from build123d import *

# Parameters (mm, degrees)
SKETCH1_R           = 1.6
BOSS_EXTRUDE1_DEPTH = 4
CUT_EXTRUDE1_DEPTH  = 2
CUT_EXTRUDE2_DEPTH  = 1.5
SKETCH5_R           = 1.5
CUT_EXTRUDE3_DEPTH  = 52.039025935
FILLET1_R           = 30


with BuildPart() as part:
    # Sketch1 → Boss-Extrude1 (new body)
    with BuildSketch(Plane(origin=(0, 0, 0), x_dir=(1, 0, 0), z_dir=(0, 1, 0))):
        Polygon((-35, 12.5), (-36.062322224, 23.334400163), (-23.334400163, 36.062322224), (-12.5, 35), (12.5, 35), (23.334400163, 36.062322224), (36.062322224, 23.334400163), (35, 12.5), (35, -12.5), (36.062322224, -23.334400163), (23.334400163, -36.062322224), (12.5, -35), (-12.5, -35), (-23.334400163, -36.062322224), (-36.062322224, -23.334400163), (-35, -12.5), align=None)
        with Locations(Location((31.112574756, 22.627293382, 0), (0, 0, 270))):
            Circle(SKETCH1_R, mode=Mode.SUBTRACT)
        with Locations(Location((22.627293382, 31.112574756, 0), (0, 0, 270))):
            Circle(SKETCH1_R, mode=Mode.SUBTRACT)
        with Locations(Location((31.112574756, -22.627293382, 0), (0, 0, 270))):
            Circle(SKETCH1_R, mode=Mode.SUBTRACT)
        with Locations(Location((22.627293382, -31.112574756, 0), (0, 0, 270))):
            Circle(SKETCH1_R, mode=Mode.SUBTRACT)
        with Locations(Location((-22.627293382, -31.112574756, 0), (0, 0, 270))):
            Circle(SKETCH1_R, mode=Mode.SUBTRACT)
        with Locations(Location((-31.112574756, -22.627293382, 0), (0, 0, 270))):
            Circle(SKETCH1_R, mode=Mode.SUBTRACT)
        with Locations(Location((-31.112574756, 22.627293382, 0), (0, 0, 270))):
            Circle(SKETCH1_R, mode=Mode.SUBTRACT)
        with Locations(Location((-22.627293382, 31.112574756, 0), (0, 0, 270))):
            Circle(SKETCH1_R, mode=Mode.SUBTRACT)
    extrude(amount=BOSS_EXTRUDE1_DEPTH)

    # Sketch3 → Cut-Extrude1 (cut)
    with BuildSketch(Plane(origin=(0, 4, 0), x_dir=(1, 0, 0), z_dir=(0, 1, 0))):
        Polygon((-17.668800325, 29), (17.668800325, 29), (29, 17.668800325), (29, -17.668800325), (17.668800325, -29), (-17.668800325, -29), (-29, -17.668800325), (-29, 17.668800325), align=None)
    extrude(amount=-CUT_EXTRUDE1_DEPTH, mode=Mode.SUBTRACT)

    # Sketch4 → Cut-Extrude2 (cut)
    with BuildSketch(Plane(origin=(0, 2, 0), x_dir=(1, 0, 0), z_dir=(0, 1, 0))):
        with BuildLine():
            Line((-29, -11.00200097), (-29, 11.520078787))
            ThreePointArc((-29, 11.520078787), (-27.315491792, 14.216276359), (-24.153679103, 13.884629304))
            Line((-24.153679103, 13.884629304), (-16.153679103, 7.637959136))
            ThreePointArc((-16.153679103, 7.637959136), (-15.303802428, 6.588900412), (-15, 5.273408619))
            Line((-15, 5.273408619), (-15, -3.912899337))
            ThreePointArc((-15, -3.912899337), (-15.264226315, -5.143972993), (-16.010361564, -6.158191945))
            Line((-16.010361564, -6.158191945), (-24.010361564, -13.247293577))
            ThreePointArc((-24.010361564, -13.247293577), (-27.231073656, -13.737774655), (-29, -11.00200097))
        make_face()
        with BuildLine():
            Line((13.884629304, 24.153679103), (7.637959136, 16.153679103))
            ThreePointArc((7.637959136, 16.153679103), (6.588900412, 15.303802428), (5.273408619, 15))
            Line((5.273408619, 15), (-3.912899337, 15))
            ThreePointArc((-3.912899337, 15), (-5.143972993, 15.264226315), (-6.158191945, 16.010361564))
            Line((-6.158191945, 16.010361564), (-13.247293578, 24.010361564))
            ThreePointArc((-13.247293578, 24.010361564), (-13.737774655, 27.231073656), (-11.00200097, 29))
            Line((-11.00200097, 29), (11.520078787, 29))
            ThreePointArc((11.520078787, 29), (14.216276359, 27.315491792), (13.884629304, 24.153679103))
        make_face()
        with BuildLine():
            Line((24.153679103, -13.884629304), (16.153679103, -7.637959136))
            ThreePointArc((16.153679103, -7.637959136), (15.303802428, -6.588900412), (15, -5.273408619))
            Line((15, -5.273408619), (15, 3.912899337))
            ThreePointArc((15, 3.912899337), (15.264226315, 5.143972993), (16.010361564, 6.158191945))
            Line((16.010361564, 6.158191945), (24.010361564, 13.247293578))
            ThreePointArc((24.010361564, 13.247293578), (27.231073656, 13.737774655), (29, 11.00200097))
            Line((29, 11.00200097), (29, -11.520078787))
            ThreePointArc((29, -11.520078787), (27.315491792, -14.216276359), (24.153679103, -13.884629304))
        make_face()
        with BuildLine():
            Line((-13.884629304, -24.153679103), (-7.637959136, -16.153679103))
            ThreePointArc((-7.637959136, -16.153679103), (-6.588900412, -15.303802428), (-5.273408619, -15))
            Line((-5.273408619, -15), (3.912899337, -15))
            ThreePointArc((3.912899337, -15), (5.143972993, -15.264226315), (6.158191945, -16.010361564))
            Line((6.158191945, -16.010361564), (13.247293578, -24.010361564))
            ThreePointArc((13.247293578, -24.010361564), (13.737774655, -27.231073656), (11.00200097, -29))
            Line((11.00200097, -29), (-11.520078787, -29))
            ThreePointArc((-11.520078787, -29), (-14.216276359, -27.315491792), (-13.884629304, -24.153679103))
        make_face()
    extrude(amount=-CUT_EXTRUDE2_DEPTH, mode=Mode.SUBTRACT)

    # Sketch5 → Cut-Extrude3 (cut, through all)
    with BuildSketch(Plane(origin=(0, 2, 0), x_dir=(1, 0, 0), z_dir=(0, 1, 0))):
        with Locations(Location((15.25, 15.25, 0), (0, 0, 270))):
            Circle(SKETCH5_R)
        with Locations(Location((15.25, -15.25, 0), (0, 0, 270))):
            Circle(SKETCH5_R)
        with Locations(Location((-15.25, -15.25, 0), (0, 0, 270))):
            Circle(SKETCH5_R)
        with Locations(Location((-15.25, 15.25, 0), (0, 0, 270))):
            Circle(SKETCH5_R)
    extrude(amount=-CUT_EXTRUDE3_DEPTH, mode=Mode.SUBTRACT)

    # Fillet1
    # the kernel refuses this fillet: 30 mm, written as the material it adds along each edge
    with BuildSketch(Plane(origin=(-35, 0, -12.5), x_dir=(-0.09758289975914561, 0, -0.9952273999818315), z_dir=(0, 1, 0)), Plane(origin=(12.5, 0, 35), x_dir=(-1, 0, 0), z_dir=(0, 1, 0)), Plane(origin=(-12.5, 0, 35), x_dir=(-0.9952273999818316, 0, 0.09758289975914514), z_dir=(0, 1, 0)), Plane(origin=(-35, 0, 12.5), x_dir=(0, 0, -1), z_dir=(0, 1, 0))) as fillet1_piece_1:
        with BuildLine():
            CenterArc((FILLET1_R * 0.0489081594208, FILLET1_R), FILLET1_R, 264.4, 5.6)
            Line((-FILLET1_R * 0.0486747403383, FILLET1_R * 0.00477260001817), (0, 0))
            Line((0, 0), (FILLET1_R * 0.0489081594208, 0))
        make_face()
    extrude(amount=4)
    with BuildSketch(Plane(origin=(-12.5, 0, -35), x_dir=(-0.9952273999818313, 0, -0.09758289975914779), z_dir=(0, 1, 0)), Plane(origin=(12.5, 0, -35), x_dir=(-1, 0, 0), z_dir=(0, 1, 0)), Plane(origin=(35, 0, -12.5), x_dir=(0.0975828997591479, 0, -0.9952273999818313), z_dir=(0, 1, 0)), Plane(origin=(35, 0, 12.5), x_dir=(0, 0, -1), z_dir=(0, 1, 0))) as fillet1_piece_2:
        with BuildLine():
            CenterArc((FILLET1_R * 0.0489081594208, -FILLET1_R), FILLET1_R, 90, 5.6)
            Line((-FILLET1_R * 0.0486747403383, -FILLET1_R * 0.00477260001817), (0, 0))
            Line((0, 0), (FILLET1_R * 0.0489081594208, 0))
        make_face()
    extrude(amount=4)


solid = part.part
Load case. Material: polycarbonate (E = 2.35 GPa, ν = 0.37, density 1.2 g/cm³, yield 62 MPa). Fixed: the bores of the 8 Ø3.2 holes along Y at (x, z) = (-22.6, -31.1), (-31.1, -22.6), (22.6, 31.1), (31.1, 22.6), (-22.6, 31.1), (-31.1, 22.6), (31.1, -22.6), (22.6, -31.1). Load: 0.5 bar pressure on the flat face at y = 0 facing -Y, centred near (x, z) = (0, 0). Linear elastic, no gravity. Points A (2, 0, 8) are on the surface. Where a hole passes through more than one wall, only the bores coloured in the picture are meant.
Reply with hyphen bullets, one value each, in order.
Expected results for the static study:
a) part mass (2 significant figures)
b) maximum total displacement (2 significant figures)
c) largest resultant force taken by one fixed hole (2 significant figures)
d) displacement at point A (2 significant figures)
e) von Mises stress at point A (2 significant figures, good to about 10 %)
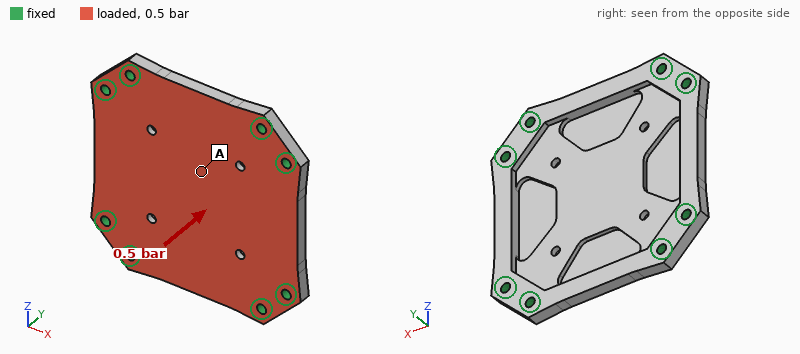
- 13 g
- 1.1 mm
- 36 N
- 1.00 mm
- 8.5 MPa
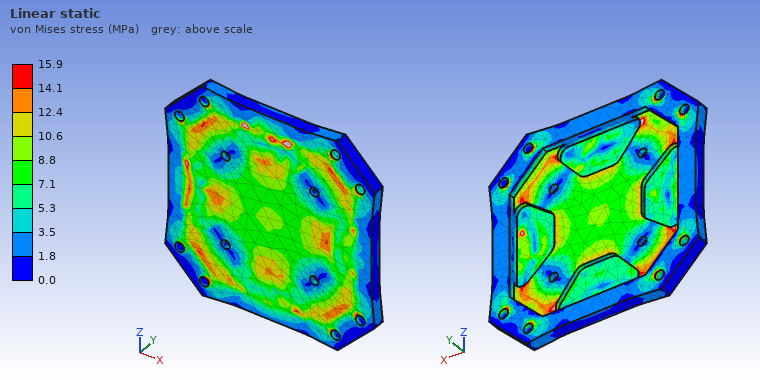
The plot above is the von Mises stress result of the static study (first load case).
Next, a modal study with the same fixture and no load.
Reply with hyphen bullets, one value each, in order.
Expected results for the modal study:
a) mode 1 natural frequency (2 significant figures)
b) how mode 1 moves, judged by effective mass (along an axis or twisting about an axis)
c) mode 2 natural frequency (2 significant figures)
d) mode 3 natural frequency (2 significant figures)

- 930 Hz
- along Y
- 1900 Hz
- 1900 Hz
